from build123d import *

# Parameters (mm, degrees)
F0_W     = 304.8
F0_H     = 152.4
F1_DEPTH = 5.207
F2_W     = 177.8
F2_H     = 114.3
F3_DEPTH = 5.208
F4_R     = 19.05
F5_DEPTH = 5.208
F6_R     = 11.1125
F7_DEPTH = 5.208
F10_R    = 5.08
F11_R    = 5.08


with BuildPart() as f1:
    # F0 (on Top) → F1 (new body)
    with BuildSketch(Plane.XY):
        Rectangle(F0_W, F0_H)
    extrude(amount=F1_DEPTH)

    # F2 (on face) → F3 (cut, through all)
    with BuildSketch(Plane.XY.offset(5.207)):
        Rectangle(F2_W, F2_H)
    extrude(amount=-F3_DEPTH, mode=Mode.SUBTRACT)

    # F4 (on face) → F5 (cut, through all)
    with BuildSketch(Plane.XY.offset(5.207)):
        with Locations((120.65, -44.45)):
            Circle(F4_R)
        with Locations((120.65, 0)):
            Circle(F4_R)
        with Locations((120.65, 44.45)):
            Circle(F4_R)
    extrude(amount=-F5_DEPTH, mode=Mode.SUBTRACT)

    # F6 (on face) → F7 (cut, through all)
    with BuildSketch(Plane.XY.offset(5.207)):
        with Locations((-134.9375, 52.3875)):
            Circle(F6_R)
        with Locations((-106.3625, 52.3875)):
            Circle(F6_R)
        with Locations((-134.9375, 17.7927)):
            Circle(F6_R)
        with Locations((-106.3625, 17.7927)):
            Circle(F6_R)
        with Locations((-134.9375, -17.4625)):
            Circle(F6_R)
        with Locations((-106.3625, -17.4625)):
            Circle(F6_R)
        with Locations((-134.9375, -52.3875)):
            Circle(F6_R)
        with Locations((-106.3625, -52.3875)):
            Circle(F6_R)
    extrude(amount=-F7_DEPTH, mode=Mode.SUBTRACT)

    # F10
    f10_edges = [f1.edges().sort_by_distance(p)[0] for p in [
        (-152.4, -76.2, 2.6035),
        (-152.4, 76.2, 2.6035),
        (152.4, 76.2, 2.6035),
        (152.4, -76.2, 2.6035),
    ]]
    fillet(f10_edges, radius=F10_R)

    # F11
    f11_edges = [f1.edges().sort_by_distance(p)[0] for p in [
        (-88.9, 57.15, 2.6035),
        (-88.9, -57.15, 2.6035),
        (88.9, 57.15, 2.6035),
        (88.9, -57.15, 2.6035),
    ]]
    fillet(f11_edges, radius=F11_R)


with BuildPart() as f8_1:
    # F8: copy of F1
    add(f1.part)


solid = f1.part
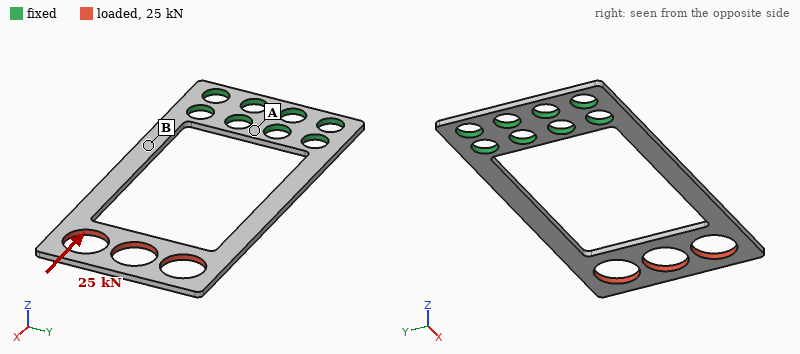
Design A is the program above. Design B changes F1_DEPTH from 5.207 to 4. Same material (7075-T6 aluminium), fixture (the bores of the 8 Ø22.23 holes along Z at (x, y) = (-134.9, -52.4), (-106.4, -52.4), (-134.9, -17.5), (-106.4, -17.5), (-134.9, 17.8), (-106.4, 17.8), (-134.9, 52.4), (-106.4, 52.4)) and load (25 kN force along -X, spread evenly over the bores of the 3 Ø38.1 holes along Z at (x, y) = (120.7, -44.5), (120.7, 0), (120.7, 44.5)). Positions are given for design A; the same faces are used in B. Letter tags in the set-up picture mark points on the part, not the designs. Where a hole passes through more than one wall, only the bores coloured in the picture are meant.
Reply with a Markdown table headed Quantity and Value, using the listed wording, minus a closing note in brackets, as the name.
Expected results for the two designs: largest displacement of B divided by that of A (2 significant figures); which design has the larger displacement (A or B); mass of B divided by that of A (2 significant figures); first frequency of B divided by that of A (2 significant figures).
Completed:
| Quantity | Value |
|---|---|
| largest displacement of B divided by that of A | 1.3 |
| which design has the larger displacement | B |
| mass of B divided by that of A | 0.77 |
| first frequency of B divided by that of A | 0.77 |
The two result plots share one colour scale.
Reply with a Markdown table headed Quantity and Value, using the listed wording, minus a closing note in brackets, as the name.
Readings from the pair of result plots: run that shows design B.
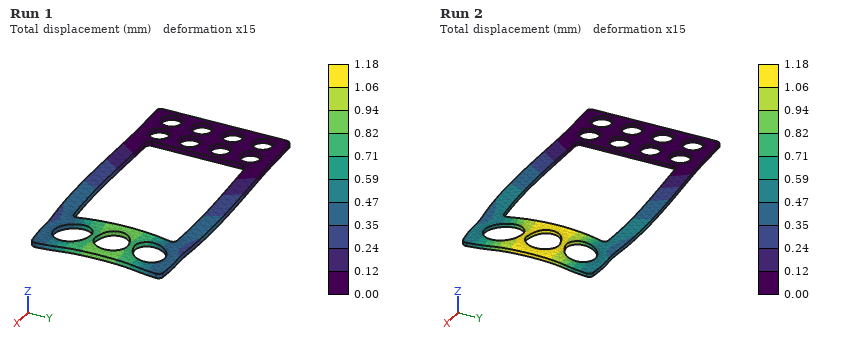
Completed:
| Quantity | Value |
|---|---|
| run that shows design B | Run 2 |
